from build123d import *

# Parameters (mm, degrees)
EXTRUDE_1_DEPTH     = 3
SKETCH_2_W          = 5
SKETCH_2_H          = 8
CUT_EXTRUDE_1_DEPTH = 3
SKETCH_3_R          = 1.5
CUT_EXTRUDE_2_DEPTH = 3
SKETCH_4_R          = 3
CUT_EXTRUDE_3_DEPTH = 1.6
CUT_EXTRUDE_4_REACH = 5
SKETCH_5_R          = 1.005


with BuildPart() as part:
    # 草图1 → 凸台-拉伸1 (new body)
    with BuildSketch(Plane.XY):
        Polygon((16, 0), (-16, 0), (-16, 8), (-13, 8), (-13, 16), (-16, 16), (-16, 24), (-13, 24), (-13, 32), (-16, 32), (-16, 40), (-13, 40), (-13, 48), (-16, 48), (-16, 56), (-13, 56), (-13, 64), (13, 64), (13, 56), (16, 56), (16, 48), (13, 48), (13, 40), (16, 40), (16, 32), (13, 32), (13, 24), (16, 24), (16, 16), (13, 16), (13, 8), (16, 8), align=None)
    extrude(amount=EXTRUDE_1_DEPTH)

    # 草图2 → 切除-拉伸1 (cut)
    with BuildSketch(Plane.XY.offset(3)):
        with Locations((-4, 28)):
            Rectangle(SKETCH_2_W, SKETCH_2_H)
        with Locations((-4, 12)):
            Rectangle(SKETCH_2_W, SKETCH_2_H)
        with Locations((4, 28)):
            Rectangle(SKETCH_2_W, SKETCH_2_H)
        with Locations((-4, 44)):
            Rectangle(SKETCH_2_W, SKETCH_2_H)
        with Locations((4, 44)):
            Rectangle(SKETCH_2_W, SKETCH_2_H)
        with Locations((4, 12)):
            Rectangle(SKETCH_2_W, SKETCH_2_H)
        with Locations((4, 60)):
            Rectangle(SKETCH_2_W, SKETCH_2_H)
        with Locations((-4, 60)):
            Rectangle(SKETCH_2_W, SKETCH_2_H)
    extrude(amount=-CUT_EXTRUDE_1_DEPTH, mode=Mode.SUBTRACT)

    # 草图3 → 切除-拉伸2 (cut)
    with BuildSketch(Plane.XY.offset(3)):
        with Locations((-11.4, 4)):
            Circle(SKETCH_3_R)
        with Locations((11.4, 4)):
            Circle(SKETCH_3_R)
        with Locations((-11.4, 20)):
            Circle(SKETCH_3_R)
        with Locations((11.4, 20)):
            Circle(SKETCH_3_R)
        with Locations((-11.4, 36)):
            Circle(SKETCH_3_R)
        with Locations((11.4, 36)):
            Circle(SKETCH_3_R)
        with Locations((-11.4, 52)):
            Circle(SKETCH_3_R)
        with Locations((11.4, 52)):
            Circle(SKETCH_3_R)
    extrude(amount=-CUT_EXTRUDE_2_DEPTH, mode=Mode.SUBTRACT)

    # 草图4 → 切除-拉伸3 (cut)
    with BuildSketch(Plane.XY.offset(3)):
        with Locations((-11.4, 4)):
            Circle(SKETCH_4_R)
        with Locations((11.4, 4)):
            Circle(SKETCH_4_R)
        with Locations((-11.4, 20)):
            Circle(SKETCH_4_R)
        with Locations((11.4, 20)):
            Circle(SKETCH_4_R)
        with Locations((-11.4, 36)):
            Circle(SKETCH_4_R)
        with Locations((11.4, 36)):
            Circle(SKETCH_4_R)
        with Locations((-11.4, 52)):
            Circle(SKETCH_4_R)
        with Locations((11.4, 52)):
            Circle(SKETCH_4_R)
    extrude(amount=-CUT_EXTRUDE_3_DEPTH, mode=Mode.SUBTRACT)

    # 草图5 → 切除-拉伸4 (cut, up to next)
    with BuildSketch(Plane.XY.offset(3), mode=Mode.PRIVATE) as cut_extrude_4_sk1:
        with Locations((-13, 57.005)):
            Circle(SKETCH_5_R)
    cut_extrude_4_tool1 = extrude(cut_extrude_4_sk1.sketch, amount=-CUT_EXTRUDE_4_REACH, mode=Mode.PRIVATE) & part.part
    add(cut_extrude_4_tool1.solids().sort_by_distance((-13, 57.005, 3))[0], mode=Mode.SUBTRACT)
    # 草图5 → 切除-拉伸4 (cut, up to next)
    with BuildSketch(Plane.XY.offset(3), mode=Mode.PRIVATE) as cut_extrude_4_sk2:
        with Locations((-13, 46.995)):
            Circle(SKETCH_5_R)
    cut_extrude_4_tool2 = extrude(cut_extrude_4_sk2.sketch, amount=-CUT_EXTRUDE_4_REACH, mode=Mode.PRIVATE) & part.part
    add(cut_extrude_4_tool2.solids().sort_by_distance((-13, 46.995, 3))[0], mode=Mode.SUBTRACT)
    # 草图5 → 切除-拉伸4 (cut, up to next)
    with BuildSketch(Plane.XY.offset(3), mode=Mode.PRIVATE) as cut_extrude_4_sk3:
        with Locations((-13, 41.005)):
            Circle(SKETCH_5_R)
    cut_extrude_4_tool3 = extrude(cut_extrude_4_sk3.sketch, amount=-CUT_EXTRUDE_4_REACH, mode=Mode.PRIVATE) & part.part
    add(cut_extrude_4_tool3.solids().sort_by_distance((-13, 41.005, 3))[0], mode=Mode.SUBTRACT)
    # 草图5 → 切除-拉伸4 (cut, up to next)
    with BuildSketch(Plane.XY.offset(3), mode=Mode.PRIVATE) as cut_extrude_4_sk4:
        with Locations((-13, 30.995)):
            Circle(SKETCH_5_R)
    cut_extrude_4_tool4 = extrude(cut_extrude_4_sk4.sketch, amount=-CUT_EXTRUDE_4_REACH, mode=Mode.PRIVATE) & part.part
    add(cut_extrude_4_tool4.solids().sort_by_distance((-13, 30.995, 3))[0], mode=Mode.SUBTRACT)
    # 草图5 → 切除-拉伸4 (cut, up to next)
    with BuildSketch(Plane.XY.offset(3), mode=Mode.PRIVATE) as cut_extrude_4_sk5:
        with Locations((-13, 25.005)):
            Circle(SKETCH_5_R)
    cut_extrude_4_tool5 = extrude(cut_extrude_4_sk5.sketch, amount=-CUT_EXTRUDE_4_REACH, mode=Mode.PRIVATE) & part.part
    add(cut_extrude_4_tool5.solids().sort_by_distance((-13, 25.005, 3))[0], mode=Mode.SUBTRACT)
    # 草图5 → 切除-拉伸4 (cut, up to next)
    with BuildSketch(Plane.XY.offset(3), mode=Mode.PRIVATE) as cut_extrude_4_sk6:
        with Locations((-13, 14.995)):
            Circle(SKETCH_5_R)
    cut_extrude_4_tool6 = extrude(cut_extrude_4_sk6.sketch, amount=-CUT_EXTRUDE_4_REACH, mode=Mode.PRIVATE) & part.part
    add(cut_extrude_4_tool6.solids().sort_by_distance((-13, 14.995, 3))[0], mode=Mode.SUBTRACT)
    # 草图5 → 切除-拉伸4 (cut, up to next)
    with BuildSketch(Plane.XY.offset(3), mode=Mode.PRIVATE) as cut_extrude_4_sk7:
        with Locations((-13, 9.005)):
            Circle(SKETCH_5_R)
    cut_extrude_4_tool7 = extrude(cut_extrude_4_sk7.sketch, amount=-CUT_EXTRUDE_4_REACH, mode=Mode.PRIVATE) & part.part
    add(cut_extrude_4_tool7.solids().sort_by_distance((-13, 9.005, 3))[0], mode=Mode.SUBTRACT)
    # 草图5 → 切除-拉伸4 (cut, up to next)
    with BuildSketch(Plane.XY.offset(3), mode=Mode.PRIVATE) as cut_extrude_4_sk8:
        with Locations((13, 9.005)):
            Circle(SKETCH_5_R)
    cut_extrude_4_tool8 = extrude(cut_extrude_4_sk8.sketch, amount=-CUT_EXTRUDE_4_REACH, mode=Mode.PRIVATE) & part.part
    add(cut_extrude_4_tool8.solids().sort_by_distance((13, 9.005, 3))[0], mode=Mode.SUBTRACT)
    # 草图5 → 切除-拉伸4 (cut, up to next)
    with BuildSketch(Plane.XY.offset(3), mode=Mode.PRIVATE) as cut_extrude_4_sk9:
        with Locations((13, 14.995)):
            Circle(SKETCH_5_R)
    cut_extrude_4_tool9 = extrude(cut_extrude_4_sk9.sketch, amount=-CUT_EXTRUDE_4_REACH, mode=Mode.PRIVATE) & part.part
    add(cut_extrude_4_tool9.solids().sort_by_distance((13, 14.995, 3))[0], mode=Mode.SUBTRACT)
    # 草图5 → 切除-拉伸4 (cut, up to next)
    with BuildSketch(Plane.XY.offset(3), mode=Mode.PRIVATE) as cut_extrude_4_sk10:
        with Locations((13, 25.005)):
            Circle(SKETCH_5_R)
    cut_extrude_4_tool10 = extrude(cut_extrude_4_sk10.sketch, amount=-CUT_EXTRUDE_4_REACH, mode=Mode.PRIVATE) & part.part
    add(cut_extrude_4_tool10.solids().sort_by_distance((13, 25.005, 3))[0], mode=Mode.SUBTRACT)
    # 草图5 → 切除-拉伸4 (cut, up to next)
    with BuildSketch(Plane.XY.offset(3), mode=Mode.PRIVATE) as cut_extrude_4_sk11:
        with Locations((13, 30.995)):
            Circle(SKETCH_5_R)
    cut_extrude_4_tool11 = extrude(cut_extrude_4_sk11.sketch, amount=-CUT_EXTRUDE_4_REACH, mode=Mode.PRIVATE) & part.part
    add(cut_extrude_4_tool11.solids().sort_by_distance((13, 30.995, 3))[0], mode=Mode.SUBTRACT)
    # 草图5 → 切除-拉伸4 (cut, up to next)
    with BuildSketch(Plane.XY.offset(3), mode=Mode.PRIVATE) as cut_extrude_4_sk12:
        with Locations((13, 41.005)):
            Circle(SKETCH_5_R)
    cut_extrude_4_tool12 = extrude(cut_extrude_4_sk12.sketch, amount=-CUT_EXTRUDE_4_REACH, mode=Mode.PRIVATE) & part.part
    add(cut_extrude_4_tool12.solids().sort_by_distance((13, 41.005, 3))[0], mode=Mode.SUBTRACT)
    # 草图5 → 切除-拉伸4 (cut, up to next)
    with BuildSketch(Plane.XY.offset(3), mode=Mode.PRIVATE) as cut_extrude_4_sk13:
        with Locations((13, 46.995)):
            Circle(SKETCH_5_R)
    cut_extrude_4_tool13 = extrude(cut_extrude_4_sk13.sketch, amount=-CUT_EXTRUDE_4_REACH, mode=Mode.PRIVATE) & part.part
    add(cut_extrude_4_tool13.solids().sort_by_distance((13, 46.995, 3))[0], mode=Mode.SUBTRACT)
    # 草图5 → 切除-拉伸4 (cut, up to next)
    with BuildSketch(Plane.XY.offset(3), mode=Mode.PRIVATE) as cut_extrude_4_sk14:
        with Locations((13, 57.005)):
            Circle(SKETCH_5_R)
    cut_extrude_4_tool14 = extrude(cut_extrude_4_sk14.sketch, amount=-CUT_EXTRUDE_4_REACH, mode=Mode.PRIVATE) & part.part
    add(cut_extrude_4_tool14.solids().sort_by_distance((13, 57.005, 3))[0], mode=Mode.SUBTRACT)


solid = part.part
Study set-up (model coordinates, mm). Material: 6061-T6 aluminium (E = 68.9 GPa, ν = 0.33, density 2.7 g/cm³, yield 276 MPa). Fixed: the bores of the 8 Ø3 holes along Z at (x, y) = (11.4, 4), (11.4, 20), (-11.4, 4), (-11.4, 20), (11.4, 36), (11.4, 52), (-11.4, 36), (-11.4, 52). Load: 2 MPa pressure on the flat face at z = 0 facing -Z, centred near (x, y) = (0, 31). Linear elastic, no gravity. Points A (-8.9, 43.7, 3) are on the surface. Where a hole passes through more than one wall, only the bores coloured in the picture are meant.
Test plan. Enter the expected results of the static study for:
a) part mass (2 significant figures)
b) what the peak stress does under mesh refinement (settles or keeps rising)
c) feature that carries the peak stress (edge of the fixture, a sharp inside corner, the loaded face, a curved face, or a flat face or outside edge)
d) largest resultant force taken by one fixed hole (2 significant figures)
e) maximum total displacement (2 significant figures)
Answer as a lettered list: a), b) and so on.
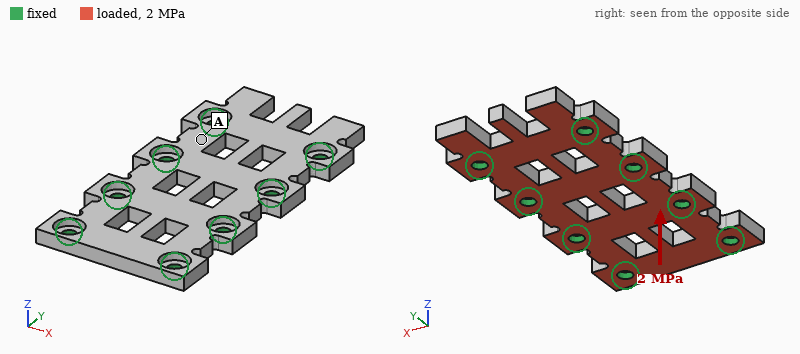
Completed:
a) 11 g
b) keeps rising
c) edge of the fixture
d) 520 N
e) 72 µm
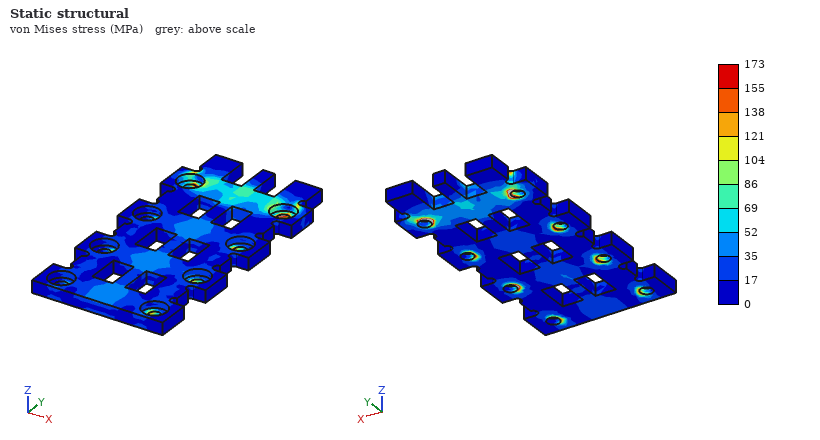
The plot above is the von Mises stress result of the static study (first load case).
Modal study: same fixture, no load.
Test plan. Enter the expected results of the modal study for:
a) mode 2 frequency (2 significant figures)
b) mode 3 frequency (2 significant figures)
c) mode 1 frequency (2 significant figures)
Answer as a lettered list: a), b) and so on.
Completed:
a) 14 kHz
b) 17 kHz
c) 12 kHz
